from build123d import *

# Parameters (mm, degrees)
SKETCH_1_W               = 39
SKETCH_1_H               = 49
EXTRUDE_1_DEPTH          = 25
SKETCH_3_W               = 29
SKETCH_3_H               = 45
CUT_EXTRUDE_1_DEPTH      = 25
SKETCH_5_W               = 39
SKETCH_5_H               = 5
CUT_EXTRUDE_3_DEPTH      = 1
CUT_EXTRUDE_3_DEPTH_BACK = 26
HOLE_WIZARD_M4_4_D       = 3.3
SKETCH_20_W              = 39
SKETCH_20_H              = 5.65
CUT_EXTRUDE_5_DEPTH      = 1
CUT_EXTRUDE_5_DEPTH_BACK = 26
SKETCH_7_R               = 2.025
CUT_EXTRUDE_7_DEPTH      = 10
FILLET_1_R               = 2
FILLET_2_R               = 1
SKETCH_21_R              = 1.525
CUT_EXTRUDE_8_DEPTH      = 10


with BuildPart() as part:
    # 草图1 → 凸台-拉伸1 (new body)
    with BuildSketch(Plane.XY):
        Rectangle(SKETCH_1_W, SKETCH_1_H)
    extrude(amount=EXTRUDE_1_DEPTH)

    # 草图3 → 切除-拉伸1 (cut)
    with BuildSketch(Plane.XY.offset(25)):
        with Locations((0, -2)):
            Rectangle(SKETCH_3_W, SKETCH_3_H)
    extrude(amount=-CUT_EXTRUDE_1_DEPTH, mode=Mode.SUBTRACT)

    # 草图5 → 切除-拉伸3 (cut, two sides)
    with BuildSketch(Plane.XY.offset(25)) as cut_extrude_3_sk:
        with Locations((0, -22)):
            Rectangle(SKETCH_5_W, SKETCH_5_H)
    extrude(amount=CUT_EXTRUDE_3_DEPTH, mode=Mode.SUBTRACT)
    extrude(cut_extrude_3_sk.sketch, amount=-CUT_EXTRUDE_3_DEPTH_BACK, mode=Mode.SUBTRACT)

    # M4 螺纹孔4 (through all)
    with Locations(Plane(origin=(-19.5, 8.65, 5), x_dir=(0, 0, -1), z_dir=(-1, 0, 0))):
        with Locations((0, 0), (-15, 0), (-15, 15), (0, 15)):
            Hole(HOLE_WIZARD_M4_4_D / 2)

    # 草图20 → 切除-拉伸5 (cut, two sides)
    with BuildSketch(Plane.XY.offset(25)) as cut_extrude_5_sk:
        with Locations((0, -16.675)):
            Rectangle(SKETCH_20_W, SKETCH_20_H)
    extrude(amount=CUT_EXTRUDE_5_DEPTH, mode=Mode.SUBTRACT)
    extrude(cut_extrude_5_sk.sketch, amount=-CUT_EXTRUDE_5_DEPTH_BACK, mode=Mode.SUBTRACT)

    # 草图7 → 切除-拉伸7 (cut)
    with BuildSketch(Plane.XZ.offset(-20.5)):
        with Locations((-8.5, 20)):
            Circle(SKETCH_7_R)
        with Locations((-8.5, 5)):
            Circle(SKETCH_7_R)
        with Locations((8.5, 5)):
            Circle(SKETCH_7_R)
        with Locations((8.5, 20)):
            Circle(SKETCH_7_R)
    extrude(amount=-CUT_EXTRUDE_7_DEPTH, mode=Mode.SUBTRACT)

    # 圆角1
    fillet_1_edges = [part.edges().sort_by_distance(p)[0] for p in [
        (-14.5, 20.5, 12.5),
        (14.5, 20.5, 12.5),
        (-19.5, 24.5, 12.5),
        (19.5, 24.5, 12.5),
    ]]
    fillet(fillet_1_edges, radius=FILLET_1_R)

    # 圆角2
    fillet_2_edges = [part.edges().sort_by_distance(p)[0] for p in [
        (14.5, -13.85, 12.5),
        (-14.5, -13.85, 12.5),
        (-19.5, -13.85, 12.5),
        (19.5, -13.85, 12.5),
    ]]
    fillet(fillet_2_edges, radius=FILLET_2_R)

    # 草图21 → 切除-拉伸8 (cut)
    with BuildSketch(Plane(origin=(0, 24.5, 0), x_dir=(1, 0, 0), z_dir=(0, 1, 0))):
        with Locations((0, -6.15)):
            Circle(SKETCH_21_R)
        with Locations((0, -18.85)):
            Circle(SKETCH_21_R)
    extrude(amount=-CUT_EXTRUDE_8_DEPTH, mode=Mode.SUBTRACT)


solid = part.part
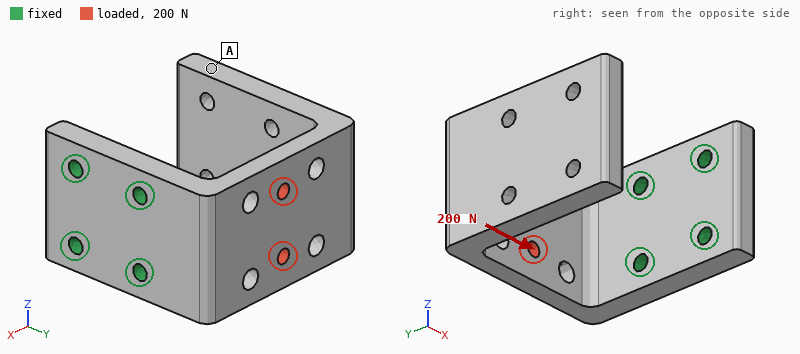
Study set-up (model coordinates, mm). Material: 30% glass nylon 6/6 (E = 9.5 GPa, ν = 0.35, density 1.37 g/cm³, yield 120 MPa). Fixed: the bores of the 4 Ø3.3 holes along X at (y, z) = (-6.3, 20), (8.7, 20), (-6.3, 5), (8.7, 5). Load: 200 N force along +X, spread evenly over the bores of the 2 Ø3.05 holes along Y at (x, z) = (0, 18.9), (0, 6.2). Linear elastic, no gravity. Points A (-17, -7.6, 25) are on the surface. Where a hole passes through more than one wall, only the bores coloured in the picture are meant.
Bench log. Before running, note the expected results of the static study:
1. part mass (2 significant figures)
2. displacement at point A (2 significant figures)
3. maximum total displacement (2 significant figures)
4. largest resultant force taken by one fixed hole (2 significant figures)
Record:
16 g
0.29 mm
0.33 mm
120 N
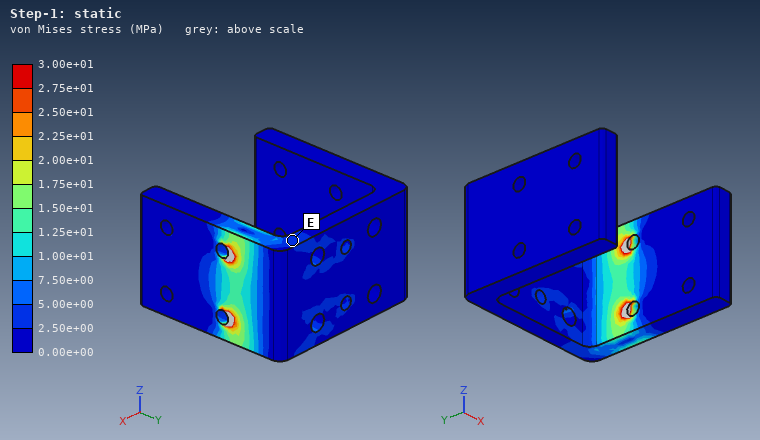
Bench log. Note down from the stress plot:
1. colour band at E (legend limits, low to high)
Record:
2.50e+00 to 5.00e+00 MPa
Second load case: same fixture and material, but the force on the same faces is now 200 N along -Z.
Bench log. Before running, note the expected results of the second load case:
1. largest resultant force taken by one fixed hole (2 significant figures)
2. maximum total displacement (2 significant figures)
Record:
260 N
0.40 mm
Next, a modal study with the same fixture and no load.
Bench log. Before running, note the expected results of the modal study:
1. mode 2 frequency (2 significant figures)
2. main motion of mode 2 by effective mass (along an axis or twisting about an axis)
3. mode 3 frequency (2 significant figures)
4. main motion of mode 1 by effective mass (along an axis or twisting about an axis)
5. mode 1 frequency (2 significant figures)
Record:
600 Hz
along Z
1100 Hz
along Y
380 Hz
